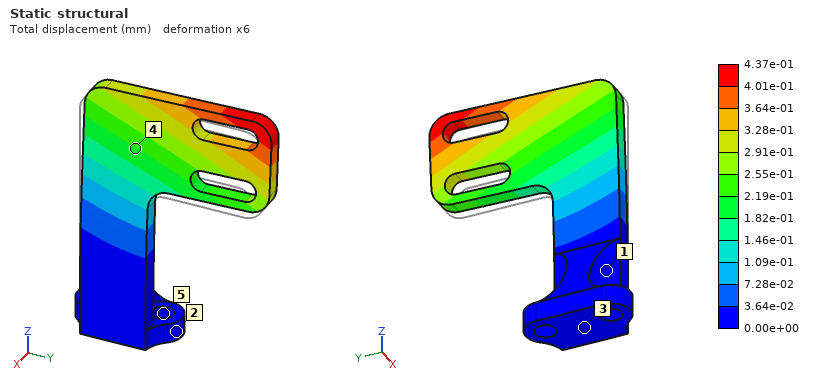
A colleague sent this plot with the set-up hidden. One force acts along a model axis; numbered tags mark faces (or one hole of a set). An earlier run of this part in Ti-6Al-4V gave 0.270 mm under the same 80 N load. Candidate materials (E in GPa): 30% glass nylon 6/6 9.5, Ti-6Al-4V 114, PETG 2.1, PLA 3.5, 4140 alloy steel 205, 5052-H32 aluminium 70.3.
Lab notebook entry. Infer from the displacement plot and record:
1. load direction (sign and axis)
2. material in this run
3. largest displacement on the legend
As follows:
-X
5052-H32 aluminium
4.37e-01 mm
